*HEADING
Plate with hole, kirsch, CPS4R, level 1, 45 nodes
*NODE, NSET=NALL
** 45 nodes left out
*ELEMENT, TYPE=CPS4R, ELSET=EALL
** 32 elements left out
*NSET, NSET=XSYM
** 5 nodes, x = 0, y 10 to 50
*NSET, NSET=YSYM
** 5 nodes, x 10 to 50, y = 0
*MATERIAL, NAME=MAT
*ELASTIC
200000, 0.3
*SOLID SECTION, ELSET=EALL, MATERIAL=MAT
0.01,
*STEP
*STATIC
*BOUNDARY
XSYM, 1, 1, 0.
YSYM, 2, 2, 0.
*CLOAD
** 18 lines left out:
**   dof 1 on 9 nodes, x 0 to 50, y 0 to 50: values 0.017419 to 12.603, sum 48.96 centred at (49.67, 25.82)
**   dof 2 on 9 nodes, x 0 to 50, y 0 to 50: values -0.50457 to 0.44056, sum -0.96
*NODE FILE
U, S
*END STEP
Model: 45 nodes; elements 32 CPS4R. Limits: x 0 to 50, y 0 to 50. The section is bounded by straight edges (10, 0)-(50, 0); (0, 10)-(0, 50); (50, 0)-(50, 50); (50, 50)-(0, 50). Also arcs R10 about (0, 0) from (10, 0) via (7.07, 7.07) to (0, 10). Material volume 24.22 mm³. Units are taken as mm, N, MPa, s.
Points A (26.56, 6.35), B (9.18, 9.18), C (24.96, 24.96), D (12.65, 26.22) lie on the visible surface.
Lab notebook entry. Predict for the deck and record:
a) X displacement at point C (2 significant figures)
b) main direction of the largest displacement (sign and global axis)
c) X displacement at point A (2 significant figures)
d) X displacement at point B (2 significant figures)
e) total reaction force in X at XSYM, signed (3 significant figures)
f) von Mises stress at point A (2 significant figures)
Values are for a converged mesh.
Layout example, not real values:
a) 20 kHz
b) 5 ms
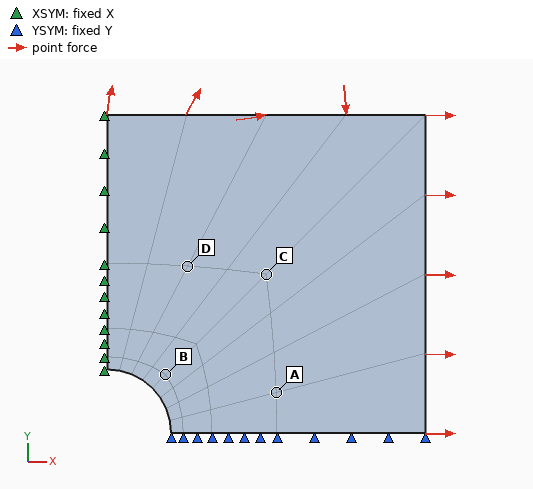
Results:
a) 0.014 mm
b) +X
c) 0.017 mm
d) 0.0092 mm
e) -49.0 N
f) 77 MPa
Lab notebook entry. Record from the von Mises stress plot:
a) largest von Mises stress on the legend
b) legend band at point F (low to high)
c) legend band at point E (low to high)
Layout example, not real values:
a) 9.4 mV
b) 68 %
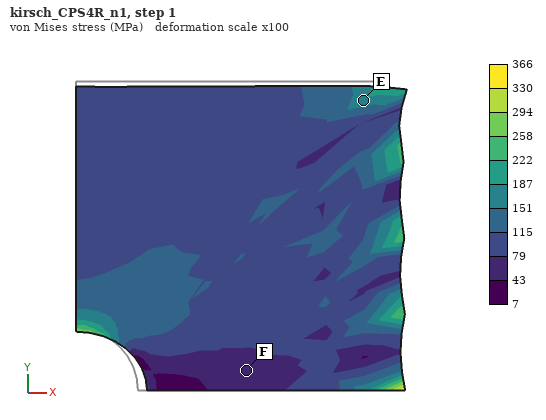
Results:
a) 366 MPa
b) 43 to 79 MPa
c) 151 to 187 MPa
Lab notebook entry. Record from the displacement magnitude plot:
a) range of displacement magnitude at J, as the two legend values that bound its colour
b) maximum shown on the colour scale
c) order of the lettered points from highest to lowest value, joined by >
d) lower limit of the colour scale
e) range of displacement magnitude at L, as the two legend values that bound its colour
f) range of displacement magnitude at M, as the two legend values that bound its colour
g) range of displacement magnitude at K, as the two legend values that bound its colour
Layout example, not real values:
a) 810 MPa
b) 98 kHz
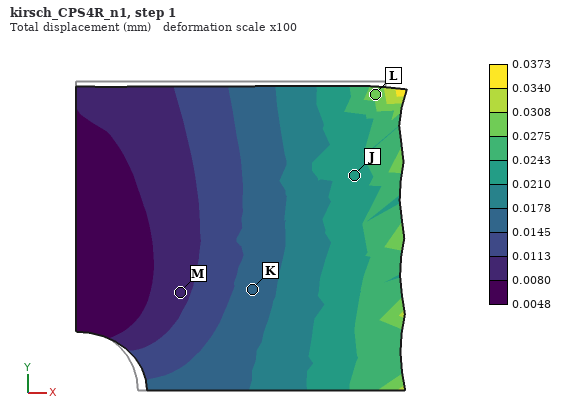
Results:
a) 0.0210 to 0.0243 mm
b) 0.0373 mm
c) L > J > K > M
d) 0.0048 mm
e) 0.0275 to 0.0308 mm
f) 0.0080 to 0.0113 mm
g) 0.0145 to 0.0178 mm
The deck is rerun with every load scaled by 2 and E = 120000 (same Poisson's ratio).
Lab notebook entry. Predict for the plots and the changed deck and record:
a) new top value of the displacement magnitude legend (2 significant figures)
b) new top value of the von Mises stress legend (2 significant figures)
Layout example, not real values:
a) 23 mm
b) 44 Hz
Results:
a) 0.12 mm
b) 730 MPa
